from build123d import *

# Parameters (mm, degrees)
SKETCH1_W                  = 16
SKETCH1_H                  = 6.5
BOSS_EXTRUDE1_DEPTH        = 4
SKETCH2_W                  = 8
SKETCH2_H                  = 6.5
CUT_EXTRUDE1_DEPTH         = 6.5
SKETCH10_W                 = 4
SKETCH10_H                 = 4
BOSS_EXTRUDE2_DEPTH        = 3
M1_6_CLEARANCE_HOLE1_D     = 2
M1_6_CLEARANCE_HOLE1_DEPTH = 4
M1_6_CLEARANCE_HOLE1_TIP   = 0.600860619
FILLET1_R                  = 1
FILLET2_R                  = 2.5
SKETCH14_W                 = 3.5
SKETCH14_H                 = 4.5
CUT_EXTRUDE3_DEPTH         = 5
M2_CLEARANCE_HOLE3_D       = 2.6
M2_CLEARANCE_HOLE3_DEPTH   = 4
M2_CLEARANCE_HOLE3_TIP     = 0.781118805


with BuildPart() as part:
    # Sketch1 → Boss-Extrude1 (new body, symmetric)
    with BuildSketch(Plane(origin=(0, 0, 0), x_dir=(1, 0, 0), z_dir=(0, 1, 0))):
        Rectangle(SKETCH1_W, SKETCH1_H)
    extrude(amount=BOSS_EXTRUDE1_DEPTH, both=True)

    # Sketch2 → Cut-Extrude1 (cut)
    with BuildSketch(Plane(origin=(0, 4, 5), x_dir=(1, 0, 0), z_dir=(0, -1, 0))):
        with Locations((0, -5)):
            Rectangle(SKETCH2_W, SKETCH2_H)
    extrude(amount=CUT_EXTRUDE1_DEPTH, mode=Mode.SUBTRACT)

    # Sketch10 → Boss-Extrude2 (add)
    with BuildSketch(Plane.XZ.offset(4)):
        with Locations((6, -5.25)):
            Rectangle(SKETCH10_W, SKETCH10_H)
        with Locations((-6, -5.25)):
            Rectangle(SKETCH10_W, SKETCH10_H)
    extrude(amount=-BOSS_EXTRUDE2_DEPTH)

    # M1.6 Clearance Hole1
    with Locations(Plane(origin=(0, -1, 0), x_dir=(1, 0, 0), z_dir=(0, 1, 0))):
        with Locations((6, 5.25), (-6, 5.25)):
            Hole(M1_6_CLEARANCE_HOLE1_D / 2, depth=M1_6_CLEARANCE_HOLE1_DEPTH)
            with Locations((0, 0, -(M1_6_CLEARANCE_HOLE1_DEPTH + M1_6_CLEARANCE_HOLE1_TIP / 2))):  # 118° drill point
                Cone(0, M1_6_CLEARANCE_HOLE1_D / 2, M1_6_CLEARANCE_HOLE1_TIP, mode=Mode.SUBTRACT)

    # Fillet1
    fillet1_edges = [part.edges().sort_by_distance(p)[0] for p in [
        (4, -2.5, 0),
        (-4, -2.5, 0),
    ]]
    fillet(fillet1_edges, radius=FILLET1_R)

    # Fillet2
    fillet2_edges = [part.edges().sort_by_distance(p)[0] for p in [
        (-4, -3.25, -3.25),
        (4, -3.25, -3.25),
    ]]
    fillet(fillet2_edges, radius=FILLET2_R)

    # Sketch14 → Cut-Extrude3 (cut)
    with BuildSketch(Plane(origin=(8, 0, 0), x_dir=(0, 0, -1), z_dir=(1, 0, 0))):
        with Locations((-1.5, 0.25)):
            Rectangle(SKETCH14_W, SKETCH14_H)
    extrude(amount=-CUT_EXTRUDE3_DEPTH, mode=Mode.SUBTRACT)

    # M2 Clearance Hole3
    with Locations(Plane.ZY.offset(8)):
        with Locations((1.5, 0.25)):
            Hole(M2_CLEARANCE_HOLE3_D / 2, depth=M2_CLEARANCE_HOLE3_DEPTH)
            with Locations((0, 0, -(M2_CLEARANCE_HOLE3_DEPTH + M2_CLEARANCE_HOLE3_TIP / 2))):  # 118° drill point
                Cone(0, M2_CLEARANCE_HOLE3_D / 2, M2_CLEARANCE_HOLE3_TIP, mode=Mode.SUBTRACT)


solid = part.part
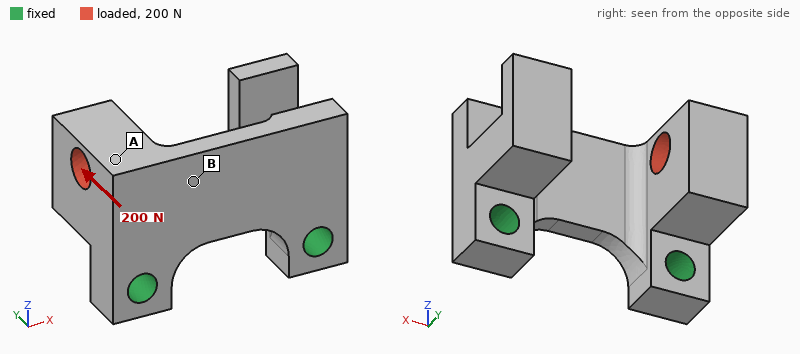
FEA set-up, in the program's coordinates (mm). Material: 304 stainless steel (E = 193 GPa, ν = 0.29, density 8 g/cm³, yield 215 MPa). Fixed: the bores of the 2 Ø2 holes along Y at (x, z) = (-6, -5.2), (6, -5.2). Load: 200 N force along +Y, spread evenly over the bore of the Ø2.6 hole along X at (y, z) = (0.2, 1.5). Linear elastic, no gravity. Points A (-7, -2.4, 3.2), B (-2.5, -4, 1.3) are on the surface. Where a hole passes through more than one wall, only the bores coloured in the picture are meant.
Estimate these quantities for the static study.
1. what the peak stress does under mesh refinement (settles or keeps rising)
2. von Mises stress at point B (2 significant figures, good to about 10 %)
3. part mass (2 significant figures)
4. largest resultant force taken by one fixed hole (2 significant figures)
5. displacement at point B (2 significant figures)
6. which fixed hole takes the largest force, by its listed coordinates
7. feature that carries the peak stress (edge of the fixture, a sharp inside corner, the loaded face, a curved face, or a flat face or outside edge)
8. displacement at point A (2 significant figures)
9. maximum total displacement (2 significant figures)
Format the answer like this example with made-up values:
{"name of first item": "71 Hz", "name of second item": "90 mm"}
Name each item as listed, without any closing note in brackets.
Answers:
{"what the peak stress does under mesh refinement": "keeps rising", "von Mises stress at point B": "33 MPa", "part mass": "4.0 g", "largest resultant force taken by one fixed hole": "190 N", "displacement at point B": "6.3 µm", "which fixed hole takes the largest force, by its listed coordinates": "(-6, -5.2)", "feature that carries the peak stress": "edge of the fixture", "displacement at point A": "11 µm", "maximum total displacement": "14 µm"}
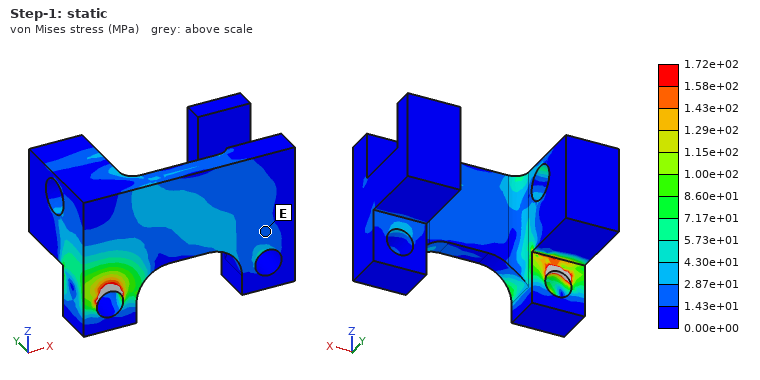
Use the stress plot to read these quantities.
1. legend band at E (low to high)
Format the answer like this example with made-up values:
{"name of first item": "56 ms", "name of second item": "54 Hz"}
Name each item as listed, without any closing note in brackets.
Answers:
{"legend band at E": "1.43e+01 to 2.87e+01 MPa"}
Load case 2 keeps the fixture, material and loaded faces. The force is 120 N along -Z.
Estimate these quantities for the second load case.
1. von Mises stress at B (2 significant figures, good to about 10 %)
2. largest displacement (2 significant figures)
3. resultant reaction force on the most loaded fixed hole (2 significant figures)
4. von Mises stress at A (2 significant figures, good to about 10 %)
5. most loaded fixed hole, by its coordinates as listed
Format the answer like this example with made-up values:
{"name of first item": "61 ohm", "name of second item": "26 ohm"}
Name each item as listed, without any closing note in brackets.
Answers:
{"von Mises stress at B": "10.0 MPa", "largest displacement": "4.6 µm", "resultant reaction force on the most loaded fixed hole": "120 N", "von Mises stress at A": "4.9 MPa", "most loaded fixed hole, by its coordinates as listed": "(-6, -5.2)"}
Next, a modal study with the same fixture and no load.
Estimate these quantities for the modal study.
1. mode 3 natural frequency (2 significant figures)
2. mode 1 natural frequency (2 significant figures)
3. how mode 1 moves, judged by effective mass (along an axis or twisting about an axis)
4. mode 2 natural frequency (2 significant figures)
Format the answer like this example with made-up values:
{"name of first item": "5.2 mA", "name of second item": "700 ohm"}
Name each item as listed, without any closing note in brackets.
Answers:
{"mode 3 natural frequency": "26 kHz", "mode 1 natural frequency": "19 kHz", "how mode 1 moves, judged by effective mass": "along Y", "mode 2 natural frequency": "22 kHz"}
